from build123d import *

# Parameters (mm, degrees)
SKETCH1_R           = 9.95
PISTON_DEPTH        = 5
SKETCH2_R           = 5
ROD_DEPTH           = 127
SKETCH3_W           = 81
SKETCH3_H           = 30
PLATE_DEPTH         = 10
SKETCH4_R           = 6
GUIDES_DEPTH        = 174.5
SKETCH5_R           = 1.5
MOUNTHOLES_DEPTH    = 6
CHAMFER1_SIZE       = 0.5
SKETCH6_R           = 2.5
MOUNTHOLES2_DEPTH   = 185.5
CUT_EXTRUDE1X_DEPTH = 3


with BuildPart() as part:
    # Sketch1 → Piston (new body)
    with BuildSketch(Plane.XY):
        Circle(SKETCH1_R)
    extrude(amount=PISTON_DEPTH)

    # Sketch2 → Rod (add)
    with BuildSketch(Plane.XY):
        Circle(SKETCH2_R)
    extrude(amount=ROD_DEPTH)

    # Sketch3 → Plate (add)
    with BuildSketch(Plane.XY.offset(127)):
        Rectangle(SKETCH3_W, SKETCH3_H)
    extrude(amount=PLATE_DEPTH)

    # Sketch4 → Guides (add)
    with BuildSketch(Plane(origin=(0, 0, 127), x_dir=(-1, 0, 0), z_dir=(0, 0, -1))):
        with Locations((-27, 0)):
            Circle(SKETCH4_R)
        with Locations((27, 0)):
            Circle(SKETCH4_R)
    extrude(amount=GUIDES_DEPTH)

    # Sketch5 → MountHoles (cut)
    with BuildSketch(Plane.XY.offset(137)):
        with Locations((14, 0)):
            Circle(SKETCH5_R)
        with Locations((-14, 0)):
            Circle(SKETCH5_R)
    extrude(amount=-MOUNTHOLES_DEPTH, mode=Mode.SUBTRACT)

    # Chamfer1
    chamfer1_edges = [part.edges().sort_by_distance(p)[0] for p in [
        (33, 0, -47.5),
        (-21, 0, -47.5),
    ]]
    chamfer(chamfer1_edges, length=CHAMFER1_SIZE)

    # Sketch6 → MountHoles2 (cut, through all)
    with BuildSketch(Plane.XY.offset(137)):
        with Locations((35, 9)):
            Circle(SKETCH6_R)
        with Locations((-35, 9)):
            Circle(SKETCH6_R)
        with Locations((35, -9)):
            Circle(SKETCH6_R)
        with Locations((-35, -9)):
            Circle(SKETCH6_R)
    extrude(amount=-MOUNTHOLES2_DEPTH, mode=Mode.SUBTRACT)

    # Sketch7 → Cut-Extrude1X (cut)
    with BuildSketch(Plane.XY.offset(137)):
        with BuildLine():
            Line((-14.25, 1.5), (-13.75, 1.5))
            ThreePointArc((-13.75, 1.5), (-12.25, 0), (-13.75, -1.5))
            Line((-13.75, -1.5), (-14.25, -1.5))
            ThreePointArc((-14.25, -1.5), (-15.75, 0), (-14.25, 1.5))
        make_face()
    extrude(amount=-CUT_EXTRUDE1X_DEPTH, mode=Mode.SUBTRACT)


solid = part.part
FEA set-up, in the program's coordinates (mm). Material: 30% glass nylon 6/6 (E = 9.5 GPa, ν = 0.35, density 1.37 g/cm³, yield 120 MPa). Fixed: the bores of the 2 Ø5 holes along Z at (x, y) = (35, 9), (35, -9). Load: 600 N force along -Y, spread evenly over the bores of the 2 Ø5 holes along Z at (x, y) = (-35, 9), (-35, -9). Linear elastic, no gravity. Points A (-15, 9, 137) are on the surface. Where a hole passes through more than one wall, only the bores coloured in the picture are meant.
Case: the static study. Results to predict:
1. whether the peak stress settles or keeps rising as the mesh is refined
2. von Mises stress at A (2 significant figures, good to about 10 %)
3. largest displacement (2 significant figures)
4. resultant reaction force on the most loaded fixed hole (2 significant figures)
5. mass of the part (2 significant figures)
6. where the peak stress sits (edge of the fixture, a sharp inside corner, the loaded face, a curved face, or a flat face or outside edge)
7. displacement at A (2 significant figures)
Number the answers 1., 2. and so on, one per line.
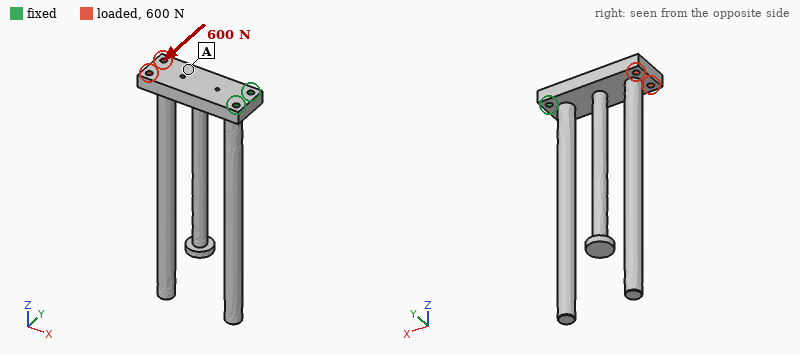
1. keeps rising
2. 6.1 MPa
3. 0.42 mm
4. 2.0 kN
5. 100 g
6. edge of the fixture
7. 0.23 mm
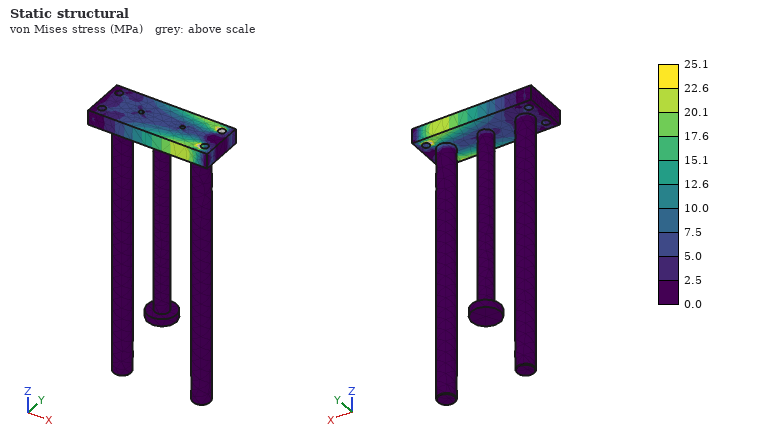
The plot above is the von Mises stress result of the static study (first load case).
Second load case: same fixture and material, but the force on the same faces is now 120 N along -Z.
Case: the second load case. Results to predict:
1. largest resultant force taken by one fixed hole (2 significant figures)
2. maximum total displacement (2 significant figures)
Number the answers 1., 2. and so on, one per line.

1. 60 N
2. 2.1 mm
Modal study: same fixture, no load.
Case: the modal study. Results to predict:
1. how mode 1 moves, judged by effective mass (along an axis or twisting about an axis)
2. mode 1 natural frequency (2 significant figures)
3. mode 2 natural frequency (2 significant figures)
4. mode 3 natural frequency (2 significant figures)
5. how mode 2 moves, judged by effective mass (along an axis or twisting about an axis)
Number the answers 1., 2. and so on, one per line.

1. along X
2. 110 Hz
3. 120 Hz
4. 140 Hz
5. along Y
